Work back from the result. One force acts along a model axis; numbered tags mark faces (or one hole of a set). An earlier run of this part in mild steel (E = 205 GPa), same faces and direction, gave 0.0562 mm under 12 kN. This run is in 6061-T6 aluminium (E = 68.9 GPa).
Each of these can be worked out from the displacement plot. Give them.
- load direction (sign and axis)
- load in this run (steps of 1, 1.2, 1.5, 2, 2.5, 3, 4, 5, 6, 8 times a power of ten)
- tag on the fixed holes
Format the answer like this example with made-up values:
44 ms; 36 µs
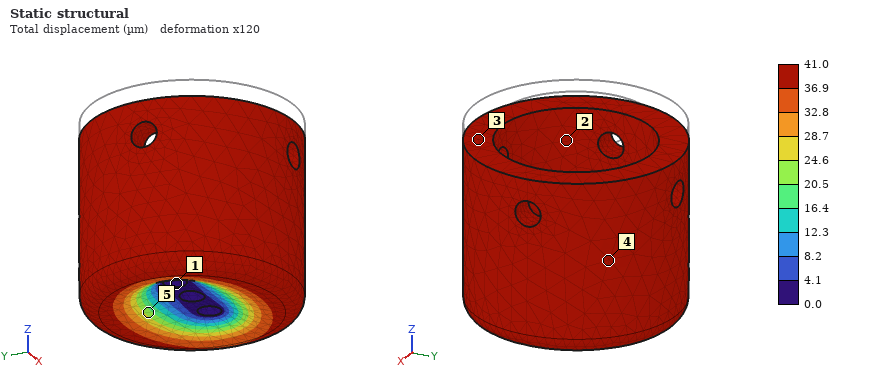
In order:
-Z; 3 kN; 1
